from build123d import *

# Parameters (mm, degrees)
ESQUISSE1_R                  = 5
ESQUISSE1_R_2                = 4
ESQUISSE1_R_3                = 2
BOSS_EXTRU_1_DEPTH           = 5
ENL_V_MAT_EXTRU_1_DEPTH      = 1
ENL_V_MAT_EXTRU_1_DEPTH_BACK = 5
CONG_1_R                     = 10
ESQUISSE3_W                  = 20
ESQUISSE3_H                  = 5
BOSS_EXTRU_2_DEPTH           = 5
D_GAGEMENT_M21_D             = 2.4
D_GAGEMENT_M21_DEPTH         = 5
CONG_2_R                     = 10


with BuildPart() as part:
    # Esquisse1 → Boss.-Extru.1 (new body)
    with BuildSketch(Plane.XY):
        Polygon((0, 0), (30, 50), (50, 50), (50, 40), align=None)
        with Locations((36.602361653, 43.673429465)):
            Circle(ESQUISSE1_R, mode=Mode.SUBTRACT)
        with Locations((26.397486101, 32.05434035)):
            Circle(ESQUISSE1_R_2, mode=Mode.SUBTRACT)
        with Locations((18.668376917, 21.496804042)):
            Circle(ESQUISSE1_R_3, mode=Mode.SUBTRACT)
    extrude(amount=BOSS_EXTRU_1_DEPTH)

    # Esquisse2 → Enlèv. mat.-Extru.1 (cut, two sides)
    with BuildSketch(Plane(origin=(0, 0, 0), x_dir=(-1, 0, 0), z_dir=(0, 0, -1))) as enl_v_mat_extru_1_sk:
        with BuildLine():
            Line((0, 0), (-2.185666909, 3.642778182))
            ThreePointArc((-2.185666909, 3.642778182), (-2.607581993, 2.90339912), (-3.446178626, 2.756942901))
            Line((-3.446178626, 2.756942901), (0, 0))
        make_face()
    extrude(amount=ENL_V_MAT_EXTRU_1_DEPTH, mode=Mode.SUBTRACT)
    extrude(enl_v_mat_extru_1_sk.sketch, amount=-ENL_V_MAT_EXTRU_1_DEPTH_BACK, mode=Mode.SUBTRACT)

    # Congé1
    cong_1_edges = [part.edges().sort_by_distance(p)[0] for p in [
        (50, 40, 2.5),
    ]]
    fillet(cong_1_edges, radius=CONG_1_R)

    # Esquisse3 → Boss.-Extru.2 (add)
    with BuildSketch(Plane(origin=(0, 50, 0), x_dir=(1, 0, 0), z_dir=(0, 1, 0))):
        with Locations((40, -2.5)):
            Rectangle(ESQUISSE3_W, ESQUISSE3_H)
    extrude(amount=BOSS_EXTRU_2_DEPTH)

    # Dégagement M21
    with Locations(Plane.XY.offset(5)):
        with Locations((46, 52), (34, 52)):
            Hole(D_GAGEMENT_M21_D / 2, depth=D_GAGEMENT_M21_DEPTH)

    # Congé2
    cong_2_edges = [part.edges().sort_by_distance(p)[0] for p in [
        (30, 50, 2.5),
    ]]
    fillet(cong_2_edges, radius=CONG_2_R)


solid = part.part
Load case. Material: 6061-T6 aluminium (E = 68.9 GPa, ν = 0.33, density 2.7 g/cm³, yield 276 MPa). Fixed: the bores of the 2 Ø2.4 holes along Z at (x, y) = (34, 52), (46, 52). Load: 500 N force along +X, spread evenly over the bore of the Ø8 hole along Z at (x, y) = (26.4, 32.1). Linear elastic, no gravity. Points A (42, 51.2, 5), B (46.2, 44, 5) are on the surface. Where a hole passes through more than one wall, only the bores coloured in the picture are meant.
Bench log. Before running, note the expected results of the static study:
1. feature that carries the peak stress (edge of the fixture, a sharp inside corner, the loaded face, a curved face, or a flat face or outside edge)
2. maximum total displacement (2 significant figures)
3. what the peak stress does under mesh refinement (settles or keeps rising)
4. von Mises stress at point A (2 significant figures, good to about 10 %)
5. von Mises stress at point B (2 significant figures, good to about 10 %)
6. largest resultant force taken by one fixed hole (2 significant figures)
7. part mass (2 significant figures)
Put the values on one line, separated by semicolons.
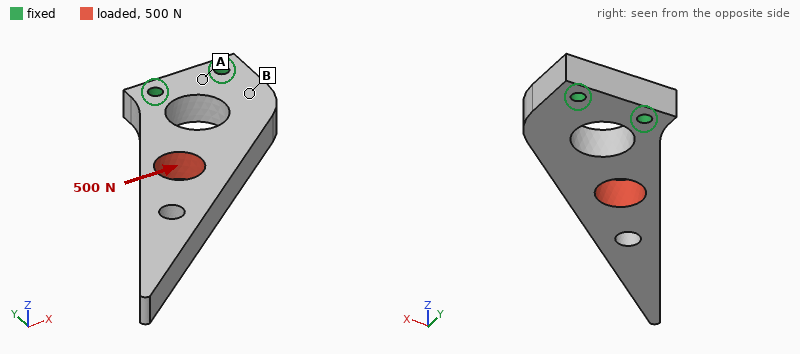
edge of the fixture; 54 µm; keeps rising; 8.4 MPa; 24 MPa; 710 N; 9.4 g
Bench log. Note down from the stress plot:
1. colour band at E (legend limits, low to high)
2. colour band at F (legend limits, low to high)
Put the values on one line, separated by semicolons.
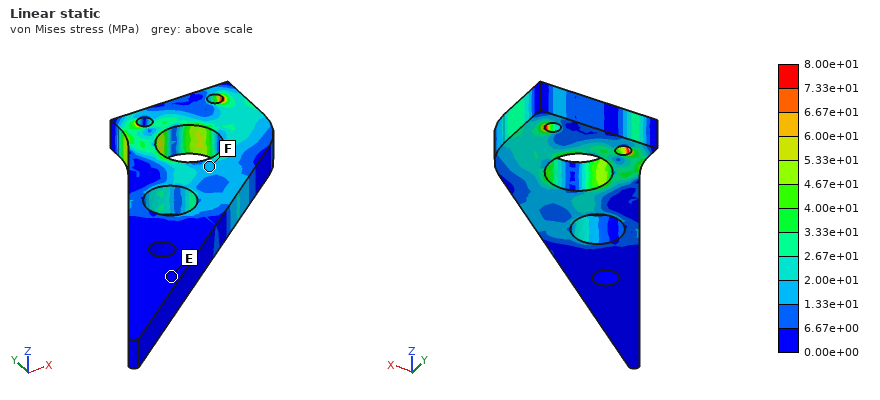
0.00e+00 to 6.67e+00 MPa; 1.33e+01 to 2.00e+01 MPa
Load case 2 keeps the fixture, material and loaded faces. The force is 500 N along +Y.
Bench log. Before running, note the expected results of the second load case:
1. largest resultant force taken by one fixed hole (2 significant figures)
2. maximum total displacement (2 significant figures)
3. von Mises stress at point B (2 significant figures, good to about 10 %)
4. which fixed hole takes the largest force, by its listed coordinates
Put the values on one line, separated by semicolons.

720 N; 40 µm; 8.8 MPa; (34, 52)
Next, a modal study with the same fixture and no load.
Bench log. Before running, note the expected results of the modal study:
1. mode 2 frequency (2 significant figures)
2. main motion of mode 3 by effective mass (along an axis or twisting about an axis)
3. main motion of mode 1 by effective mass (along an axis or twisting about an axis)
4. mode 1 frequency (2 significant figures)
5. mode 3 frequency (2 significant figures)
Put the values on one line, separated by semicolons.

5400 Hz; along Z; along Z; 1600 Hz; 7000 Hz
